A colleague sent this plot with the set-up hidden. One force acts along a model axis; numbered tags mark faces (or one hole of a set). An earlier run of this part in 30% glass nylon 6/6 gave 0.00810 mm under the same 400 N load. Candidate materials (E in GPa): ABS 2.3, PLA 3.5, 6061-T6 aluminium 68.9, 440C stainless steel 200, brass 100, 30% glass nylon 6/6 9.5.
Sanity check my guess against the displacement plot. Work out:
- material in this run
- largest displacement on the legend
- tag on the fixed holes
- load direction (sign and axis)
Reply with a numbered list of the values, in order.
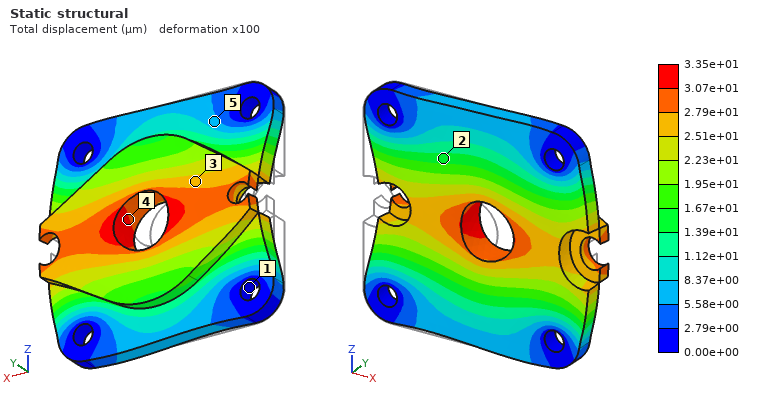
1. ABS
2. 3.35e+01 µm
3. 1
4. +X
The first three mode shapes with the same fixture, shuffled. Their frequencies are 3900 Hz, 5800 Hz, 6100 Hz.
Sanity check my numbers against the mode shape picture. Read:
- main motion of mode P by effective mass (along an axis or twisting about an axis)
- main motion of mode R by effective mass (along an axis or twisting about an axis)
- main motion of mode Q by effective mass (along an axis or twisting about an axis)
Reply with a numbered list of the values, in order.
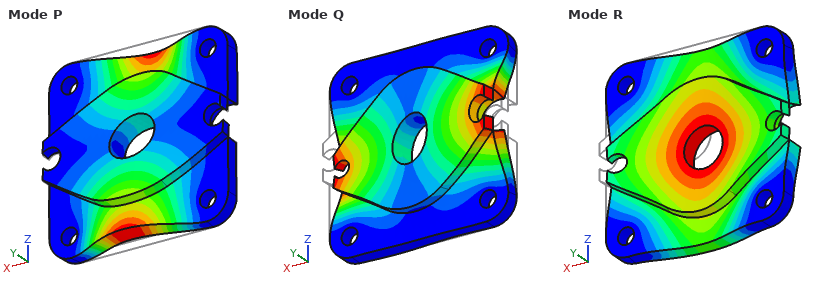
1. twisting about X
2. along Y
3. twisting about Z
